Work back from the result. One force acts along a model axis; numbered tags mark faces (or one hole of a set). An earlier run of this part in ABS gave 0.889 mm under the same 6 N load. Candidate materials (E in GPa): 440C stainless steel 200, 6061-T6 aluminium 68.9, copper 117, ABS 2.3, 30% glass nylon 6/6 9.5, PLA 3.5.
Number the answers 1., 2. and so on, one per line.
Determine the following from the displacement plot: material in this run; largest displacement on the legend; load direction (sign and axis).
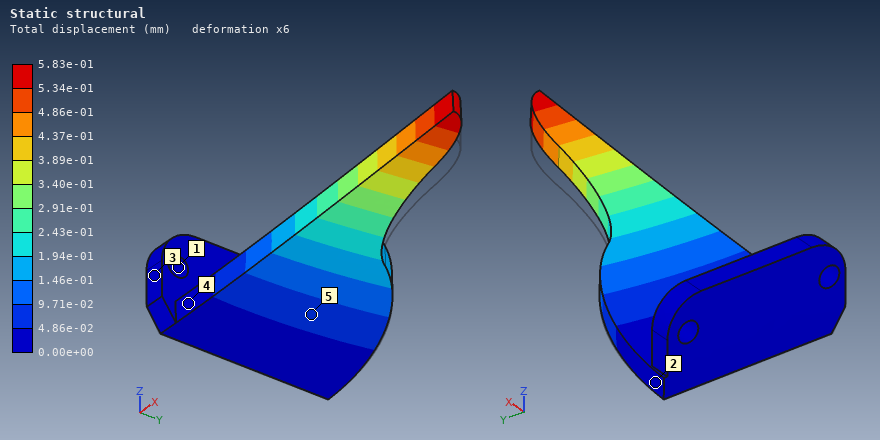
1. PLA
2. 5.83e-01 mm
3. +Z
